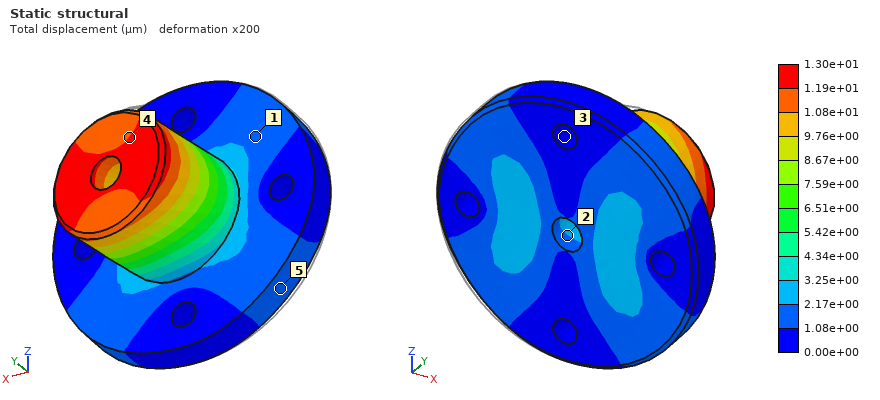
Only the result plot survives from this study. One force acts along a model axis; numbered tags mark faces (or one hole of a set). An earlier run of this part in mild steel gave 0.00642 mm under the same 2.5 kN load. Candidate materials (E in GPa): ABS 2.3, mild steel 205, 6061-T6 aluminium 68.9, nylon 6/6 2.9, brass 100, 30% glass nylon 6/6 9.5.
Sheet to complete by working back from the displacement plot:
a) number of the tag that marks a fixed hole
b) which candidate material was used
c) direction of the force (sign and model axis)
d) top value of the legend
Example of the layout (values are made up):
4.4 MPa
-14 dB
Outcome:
3
brass
+X
1.30e+01 µm
